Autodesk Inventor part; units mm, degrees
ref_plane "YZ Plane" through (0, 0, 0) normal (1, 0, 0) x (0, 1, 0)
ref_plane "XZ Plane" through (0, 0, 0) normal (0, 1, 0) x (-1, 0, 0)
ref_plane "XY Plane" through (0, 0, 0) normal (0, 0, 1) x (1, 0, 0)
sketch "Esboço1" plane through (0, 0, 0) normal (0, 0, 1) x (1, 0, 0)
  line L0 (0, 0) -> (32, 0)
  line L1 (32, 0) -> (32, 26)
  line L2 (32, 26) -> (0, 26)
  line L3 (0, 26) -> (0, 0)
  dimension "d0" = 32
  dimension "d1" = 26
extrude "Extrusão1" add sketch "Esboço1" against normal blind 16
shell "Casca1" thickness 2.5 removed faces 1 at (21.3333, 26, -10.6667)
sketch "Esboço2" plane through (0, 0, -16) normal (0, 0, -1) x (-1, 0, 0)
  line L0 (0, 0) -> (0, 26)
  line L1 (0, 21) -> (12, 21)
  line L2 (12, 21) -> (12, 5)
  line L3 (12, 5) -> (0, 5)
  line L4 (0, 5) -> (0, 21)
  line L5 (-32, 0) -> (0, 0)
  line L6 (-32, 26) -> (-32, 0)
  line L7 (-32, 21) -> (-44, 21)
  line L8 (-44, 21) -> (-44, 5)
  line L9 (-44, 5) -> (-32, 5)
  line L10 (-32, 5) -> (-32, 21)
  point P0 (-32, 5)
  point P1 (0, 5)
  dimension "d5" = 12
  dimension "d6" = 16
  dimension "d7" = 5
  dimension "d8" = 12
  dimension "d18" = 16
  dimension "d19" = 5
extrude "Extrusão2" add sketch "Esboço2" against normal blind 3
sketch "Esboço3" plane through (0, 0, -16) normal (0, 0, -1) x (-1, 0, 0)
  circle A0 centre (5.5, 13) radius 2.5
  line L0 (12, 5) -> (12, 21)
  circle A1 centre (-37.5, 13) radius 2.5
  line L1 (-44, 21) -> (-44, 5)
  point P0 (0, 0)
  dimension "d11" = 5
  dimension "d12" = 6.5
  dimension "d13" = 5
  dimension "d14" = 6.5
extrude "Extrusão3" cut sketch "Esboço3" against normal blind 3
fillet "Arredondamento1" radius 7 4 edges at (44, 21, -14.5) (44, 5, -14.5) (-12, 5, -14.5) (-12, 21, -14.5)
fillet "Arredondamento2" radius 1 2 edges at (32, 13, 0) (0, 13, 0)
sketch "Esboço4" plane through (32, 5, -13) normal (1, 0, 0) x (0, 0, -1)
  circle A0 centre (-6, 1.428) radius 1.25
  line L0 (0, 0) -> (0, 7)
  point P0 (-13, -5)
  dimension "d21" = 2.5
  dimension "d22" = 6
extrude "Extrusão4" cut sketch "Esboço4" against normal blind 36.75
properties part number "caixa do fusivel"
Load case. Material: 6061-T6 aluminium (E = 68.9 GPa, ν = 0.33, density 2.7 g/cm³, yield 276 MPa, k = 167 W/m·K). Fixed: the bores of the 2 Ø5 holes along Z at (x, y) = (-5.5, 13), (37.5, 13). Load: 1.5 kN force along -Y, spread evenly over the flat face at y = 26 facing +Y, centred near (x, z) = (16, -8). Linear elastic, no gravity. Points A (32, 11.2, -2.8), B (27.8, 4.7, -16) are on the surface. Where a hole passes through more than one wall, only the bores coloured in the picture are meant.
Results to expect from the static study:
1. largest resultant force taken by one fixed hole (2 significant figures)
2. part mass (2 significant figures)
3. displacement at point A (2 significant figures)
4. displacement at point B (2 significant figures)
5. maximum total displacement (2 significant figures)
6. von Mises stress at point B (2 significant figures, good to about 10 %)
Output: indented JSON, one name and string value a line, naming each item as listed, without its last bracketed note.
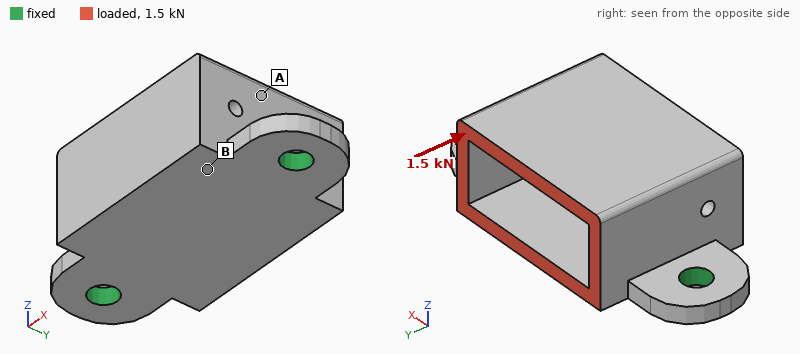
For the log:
{
  "largest resultant force taken by one fixed hole": "750 N",
  "part mass": "19 g",
  "displacement at point A": "63 µm",
  "displacement at point B": "39 µm",
  "maximum total displacement": "99 µm",
  "von Mises stress at point B": "29 MPa"
}
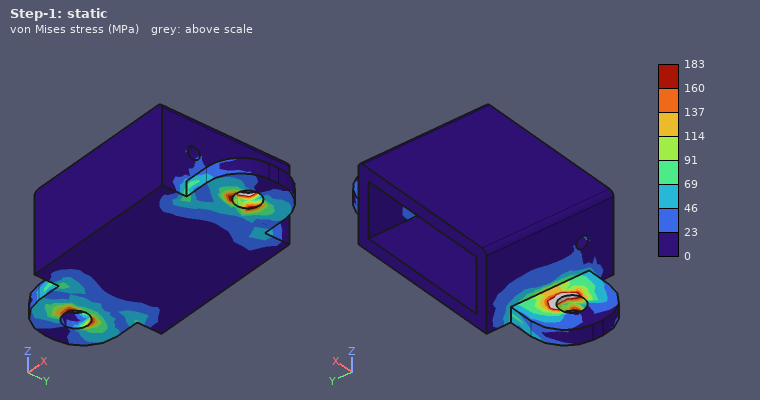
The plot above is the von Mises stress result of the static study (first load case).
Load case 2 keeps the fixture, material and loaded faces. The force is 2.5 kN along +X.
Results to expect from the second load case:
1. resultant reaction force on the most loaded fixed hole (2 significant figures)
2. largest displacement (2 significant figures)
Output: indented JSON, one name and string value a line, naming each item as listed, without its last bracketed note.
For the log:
{
  "resultant reaction force on the most loaded fixed hole": "1.5 kN",
  "largest displacement": "0.16 mm"
}
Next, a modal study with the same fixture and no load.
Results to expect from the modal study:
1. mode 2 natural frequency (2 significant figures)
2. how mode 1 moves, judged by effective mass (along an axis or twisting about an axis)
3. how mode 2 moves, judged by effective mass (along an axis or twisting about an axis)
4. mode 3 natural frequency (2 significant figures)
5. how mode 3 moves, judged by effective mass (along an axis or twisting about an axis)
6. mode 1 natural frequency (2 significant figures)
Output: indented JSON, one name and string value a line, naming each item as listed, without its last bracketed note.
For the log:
{
  "mode 2 natural frequency": "7600 Hz",
  "how mode 1 moves, judged by effective mass": "along Y",
  "how mode 2 moves, judged by effective mass": "along X",
  "mode 3 natural frequency": "10 kHz",
  "how mode 3 moves, judged by effective mass": "along Z",
  "mode 1 natural frequency": "4500 Hz"
}
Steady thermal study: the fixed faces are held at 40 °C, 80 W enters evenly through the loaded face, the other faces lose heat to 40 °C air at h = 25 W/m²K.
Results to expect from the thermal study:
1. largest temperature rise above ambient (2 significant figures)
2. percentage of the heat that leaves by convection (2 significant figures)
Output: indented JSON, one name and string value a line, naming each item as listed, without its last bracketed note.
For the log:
{
  "largest temperature rise above ambient": "75 K",
  "percentage of the heat that leaves by convection": "7.0 %"
}
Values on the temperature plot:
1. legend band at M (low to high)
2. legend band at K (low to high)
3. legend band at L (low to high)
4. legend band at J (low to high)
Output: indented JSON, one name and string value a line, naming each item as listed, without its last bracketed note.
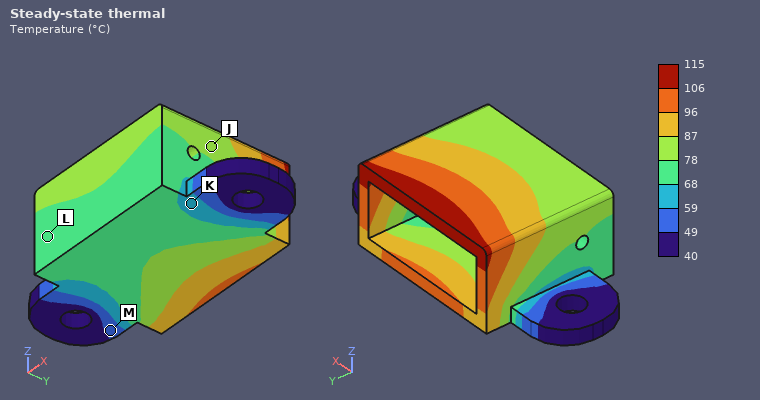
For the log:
{
  "legend band at M": "49 to 59 °C",
  "legend band at K": "59 to 68 °C",
  "legend band at L": "68 to 78 °C",
  "legend band at J": "78 to 87 °C"
}
